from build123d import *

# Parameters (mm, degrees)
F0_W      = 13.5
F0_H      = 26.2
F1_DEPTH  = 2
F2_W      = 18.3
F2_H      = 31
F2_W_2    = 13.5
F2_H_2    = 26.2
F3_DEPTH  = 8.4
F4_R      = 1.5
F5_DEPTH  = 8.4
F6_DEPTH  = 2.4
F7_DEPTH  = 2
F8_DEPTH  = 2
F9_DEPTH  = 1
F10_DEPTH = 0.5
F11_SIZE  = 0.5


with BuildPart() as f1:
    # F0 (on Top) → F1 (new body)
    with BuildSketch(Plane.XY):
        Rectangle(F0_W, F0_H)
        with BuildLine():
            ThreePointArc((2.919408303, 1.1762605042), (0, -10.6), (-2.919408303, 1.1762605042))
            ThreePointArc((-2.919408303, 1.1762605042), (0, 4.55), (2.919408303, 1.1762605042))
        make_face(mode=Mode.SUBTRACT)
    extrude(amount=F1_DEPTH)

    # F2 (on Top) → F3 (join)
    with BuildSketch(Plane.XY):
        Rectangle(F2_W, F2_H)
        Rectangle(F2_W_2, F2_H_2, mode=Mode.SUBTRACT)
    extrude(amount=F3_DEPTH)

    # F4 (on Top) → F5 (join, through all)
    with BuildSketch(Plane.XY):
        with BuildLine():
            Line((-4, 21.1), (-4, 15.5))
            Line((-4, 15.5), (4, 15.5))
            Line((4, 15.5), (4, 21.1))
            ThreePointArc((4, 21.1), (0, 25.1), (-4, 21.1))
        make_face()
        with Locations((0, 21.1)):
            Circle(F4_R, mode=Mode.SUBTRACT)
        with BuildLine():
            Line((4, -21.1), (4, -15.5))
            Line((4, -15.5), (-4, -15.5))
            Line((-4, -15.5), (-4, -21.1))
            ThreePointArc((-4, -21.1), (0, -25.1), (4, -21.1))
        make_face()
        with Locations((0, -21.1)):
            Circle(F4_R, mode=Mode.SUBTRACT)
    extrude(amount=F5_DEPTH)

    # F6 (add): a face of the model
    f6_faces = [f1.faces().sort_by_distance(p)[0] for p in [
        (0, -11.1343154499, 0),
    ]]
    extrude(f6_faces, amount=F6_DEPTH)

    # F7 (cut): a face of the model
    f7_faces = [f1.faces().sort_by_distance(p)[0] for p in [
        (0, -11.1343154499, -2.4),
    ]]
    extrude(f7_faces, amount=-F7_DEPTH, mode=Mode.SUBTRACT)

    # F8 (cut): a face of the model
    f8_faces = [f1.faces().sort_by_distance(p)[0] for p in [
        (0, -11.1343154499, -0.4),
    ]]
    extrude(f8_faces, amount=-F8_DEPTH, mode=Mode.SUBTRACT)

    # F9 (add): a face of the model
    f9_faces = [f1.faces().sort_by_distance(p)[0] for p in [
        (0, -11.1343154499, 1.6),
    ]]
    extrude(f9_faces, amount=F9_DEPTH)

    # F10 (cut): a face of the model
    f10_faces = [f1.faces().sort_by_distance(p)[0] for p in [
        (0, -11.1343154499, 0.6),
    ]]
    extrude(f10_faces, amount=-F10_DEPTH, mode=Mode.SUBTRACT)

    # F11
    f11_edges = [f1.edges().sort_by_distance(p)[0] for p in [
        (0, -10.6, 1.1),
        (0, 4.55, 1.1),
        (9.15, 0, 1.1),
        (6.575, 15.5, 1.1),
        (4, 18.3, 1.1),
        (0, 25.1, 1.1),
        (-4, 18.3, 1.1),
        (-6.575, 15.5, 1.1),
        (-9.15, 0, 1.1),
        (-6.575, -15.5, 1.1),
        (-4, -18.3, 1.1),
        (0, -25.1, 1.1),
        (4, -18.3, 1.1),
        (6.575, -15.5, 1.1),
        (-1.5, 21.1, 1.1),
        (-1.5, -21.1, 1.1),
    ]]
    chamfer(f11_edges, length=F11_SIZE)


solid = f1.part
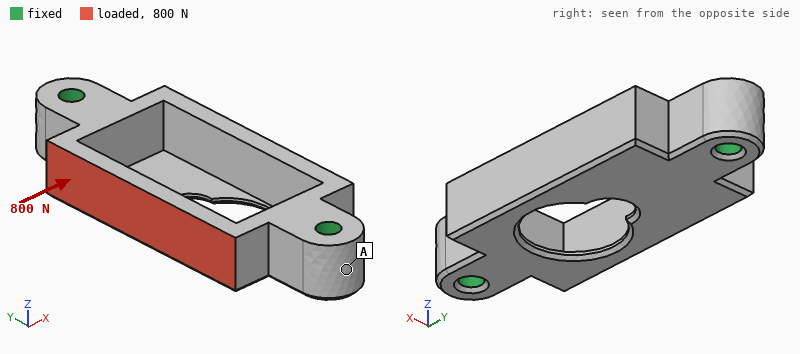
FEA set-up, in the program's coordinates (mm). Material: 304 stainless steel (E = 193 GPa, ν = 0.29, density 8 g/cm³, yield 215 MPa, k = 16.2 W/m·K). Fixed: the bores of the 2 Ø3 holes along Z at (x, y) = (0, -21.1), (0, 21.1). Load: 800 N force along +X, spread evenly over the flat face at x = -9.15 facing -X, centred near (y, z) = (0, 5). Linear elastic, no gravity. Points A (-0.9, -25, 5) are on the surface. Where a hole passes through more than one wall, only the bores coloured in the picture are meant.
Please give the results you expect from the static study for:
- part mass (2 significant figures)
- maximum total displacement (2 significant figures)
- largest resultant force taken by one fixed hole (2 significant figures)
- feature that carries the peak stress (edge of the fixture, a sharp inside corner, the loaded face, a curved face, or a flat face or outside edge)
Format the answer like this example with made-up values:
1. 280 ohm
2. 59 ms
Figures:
1. 21 g
2. 24 µm
3. 490 N
4. a curved face
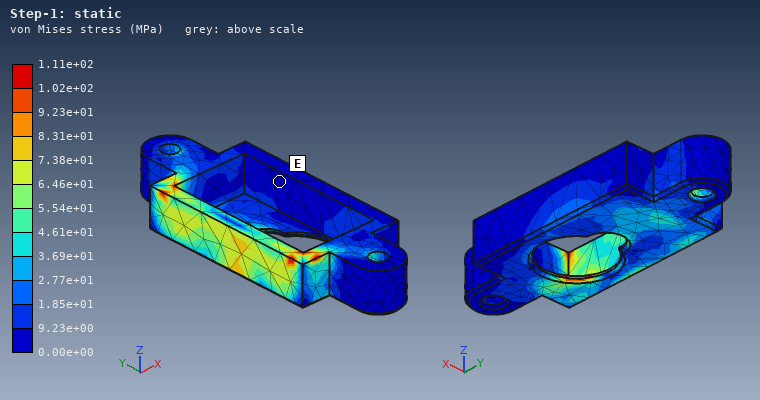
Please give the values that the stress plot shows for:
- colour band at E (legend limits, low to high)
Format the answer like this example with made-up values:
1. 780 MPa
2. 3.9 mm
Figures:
1. 0.00e+00 to 9.23e+00 MPa
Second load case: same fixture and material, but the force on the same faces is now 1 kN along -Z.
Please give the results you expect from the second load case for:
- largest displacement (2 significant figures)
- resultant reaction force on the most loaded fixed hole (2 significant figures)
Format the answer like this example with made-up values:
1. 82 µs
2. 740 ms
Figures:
1. 32 µm
2. 510 N
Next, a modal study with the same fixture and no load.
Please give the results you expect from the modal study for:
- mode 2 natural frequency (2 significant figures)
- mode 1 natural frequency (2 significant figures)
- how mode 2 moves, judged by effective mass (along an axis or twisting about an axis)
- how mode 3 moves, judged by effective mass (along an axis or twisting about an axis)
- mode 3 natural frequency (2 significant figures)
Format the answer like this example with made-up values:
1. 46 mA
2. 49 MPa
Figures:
1. 16 kHz
2. 15 kHz
3. along Z
4. along X
5. 18 kHz
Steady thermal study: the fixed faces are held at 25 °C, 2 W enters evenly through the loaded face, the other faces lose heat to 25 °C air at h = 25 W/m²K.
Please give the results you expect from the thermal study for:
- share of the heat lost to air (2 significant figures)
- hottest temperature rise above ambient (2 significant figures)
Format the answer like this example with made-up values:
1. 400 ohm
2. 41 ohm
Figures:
1. 23 %
2. 30 K
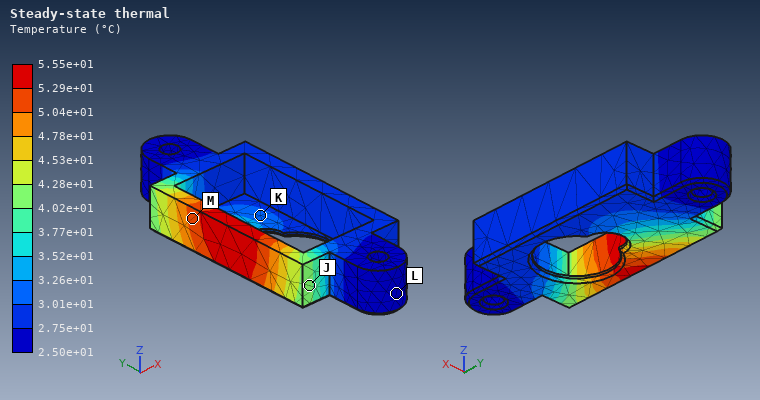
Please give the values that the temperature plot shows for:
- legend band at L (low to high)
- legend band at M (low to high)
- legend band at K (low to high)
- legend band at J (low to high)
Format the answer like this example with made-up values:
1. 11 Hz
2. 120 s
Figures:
1. 2.50e+01 to 2.75e+01 °C
2. 5.04e+01 to 5.29e+01 °C
3. 3.01e+01 to 3.26e+01 °C
4. 4.02e+01 to 4.28e+01 °C
